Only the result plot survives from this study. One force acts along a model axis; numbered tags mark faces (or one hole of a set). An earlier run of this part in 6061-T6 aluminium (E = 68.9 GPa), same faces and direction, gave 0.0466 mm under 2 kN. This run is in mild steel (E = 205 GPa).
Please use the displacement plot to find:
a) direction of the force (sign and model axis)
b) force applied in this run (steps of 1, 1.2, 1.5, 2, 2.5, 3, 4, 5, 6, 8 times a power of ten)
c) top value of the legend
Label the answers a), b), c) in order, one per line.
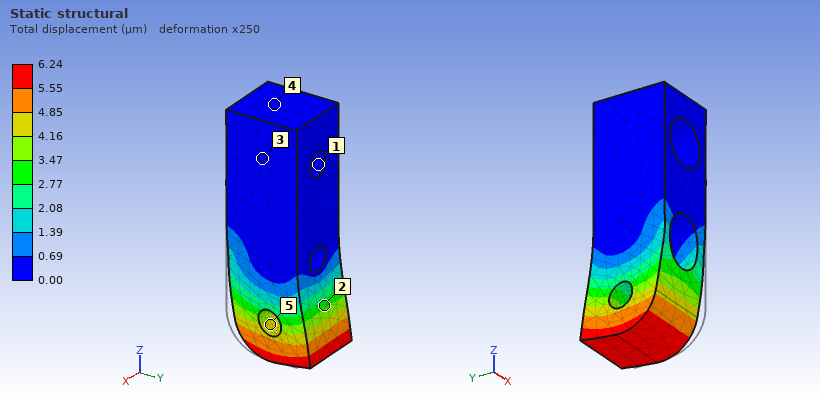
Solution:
a) +Y
b) 800 N
c) 6.24 µm
